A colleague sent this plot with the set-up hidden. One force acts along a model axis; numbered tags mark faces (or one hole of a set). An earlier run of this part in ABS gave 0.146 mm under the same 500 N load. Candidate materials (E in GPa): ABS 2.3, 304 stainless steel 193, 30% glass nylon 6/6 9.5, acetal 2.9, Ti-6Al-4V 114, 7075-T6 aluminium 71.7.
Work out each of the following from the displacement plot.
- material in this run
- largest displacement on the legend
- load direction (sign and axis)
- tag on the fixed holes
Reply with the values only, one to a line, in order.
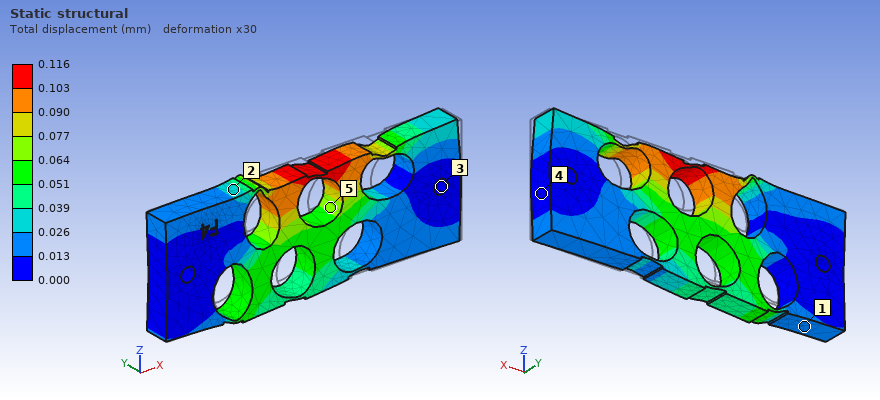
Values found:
acetal
0.116 mm
-X
3
